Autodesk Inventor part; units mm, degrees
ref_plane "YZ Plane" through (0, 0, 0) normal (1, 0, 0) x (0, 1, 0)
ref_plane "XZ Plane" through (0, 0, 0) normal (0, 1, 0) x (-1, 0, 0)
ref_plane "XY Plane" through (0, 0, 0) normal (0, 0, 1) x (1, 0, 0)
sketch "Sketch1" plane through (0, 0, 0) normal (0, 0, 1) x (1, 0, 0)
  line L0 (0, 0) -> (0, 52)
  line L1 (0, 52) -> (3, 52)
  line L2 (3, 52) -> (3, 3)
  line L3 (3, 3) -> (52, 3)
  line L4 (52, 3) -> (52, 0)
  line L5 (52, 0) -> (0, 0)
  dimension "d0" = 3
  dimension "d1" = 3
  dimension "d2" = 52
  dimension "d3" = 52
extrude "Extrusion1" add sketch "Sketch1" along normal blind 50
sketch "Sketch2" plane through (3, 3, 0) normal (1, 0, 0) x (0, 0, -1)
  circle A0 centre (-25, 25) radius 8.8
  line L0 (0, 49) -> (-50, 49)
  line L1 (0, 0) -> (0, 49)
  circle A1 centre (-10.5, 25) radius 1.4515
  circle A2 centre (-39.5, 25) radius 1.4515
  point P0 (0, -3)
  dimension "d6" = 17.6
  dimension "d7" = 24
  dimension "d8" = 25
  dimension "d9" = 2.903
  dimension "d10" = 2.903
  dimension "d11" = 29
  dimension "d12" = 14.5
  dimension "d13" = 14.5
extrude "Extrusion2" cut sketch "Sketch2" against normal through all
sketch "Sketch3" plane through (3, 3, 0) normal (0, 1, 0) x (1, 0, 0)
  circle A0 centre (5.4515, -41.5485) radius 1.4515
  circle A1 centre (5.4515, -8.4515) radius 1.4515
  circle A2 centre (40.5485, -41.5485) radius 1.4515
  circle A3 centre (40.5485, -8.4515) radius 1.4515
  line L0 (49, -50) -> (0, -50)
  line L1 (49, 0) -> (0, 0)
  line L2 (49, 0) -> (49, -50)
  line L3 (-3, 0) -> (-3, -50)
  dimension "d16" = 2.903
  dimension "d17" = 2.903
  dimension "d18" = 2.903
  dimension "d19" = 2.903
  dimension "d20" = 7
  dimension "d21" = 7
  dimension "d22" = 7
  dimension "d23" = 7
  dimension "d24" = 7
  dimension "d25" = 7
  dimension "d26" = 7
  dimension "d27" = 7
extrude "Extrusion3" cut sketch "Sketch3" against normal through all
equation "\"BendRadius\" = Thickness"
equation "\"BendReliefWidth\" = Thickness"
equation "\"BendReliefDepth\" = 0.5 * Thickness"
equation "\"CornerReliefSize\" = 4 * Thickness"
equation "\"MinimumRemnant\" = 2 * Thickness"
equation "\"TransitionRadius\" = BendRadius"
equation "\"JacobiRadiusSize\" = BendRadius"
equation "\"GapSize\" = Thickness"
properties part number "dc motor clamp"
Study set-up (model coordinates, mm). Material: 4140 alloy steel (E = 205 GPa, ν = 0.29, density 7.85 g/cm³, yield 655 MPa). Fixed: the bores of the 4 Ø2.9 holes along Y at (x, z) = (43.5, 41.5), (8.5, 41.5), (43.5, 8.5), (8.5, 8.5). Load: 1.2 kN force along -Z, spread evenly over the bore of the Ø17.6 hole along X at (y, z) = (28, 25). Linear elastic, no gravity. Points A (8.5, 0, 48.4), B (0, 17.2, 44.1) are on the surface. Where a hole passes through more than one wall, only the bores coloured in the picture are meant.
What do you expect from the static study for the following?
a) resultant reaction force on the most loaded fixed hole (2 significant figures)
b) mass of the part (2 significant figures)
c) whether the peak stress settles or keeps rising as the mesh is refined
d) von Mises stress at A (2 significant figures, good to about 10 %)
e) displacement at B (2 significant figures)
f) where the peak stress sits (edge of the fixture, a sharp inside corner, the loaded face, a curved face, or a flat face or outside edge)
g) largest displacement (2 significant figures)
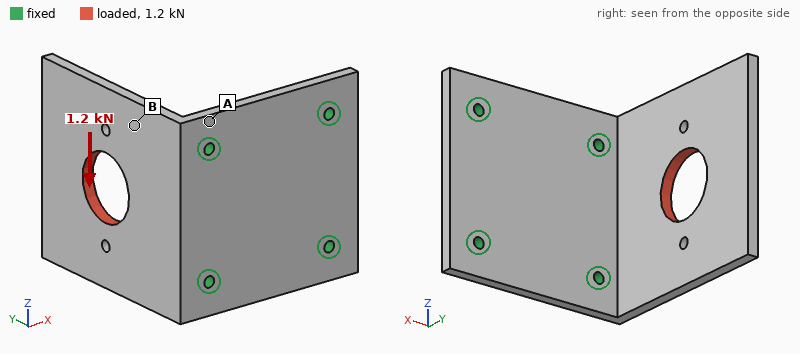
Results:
1.1 kN
110 g
keeps rising
72 MPa
26 µm
edge of the fixture
59 µm
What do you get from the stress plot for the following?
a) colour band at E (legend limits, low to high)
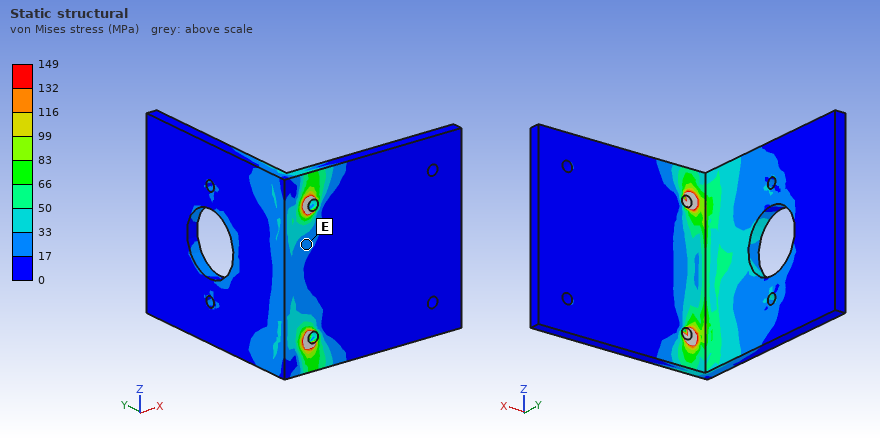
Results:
17 to 33 MPa
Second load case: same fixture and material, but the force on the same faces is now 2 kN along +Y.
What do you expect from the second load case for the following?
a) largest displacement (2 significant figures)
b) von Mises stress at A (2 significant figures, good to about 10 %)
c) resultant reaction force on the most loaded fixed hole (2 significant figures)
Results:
0.14 mm
79 MPa
1.1 kN
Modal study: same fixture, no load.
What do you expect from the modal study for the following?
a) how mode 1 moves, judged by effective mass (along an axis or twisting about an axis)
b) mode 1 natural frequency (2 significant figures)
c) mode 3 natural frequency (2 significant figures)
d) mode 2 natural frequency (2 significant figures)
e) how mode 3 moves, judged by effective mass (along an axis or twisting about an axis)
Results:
along X
790 Hz
4200 Hz
2000 Hz
along Z
